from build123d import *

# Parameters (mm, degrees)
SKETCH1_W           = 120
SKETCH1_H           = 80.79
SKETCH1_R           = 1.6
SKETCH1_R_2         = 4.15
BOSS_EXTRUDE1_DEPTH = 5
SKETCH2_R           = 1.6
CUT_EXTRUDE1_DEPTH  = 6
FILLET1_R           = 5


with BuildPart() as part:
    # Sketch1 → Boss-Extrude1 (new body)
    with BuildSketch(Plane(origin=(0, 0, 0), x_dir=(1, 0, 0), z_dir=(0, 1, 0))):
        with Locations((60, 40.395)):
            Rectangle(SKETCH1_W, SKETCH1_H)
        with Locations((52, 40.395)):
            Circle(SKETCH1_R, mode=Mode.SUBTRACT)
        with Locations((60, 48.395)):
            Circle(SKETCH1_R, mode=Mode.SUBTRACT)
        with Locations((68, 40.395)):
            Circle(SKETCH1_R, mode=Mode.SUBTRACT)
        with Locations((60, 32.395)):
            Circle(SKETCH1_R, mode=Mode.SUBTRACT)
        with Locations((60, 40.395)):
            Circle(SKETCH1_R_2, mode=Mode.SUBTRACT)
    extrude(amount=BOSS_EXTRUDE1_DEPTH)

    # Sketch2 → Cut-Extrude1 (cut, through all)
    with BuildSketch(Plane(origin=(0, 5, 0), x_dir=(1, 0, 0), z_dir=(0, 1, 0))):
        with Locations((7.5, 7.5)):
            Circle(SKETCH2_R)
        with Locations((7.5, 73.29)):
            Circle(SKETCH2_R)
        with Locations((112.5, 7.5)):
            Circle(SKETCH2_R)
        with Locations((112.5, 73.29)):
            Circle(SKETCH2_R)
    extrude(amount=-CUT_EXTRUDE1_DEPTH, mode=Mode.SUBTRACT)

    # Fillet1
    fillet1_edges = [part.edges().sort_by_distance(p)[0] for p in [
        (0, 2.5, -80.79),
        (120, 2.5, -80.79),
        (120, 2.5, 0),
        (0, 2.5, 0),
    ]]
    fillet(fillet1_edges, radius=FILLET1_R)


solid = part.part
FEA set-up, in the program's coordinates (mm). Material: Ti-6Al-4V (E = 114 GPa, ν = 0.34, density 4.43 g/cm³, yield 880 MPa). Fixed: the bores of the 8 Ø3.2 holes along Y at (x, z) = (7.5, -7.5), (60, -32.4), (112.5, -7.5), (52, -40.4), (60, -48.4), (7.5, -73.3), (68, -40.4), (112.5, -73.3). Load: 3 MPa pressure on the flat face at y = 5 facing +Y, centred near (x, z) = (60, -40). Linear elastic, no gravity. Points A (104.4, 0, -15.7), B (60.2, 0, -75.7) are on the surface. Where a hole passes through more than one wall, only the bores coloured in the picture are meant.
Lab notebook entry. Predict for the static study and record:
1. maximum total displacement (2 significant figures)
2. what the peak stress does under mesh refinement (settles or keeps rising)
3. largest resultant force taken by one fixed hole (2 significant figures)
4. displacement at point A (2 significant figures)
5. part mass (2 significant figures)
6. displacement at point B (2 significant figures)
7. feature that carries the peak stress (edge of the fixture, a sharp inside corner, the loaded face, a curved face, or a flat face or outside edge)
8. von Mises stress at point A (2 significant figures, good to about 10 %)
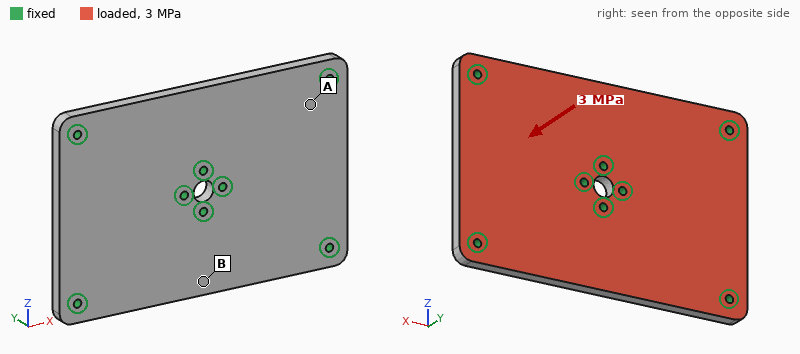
0.26 mm
keeps rising
4.0 kN
0.060 mm
210 g
0.22 mm
edge of the fixture
110 MPa
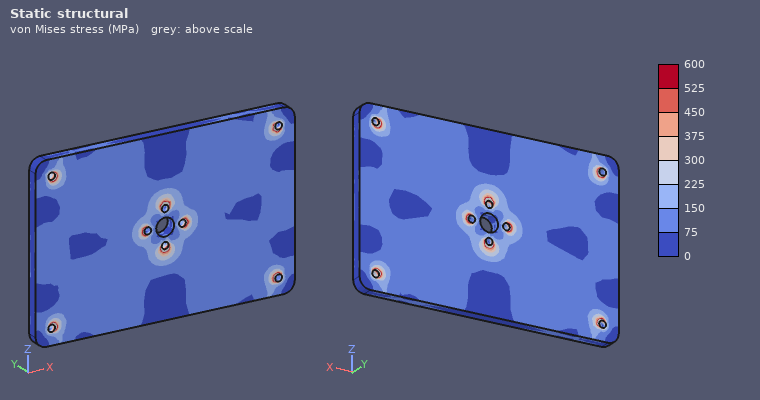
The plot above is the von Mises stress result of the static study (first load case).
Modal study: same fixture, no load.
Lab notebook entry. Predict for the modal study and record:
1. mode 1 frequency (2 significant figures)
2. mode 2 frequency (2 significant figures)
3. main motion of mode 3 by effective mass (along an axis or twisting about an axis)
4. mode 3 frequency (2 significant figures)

4500 Hz
4600 Hz
twisting about Z
5800 Hz
